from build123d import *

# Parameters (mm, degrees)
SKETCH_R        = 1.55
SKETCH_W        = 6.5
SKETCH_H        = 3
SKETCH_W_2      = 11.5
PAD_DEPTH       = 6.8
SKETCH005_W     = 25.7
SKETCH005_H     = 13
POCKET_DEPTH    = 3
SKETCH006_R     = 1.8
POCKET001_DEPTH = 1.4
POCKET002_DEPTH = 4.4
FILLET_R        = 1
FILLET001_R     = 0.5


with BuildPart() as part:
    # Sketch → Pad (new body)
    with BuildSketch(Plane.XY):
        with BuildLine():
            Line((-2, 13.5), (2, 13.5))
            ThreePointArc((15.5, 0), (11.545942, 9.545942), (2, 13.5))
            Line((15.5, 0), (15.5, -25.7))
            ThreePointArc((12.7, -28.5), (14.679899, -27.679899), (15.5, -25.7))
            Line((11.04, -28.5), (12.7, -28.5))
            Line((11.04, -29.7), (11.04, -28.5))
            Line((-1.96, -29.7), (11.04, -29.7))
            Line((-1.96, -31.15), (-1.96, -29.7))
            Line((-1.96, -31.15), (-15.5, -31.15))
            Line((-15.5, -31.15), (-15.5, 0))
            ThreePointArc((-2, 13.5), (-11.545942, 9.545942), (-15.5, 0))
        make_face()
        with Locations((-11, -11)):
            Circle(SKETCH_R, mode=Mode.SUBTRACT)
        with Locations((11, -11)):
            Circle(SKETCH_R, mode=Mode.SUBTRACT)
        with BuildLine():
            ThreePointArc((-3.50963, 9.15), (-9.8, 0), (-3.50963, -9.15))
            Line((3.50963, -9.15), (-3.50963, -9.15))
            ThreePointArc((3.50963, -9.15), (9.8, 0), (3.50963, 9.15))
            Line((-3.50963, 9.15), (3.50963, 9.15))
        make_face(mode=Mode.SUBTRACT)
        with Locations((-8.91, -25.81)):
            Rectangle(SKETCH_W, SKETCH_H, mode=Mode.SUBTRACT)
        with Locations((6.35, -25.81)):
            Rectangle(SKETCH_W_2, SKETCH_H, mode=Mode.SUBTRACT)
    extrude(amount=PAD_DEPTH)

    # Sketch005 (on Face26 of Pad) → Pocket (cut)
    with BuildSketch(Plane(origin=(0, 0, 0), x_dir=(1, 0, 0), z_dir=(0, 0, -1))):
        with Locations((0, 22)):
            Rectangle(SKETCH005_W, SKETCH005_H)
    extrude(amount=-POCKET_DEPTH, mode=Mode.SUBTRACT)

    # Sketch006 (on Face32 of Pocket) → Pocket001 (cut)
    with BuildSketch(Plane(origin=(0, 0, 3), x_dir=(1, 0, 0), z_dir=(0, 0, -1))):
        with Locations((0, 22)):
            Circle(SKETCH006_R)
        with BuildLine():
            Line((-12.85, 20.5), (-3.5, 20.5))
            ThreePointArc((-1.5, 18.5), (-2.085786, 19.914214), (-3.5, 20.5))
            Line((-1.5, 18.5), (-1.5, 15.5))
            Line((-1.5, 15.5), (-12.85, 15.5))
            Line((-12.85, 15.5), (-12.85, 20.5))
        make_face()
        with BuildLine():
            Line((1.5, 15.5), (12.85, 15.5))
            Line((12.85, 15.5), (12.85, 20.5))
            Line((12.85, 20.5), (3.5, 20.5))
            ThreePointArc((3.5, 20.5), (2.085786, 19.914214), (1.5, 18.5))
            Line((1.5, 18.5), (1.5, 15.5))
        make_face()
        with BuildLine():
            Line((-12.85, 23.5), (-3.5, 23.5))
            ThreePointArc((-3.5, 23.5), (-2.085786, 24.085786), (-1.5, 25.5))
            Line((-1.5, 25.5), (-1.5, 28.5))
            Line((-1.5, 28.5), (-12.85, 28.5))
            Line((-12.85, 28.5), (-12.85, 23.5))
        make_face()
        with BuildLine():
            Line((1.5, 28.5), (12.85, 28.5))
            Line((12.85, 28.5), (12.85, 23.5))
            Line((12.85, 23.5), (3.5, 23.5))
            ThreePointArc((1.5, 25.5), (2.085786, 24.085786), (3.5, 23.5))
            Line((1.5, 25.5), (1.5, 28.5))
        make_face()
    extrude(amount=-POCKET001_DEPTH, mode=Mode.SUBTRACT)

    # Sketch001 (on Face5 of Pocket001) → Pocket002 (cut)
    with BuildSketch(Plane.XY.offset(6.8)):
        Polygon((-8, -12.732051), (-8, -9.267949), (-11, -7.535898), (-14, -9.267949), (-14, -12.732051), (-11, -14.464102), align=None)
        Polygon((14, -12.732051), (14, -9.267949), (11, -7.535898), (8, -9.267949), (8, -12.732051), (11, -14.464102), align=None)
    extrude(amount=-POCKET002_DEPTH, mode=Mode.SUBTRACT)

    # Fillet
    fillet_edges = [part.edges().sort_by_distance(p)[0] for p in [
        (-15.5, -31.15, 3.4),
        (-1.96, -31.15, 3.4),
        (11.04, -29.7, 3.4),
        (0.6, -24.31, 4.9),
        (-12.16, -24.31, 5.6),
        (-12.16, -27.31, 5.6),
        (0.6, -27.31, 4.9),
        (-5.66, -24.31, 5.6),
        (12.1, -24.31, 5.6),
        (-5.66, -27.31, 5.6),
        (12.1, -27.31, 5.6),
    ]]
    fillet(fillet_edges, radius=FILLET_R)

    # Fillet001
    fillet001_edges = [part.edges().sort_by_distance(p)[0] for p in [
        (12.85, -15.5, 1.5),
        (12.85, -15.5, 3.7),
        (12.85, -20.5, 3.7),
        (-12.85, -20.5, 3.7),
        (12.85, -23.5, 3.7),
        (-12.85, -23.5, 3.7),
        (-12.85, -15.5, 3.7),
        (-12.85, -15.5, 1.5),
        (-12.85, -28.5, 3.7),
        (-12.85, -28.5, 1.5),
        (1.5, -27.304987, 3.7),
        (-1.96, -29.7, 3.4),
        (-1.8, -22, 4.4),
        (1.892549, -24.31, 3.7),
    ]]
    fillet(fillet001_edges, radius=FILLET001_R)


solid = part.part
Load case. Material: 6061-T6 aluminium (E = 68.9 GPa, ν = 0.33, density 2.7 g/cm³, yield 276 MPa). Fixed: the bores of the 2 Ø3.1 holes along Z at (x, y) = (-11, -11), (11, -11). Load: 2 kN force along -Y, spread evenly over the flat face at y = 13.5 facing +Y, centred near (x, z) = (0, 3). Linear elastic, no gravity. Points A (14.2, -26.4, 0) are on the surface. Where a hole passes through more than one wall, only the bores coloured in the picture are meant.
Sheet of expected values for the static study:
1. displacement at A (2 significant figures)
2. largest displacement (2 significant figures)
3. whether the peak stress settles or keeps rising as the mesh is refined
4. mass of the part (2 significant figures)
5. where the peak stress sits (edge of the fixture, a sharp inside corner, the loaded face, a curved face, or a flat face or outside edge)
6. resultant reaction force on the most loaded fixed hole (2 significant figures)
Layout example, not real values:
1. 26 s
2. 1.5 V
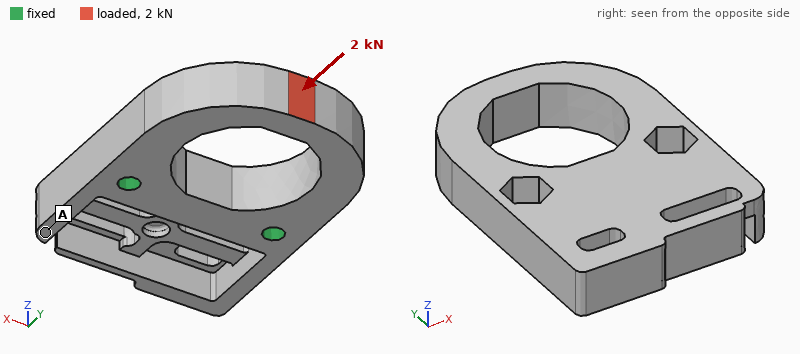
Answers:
1. 27 µm
2. 99 µm
3. keeps rising
4. 13 g
5. edge of the fixture
6. 1.1 kN
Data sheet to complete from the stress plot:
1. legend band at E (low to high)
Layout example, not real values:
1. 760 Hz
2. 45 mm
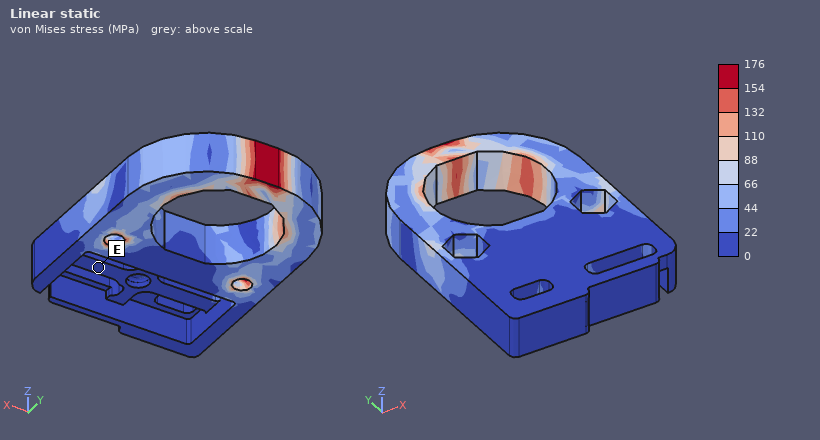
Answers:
1. 0 to 22 MPa
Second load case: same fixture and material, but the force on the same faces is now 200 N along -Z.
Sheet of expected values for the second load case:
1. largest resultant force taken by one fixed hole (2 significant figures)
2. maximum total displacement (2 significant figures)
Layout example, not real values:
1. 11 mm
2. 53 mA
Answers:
1. 100 N
2. 0.11 mm
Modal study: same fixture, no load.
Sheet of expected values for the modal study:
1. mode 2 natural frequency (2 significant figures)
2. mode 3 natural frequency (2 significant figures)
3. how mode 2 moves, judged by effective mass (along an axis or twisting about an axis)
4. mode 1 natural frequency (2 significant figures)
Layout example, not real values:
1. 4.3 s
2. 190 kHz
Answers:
1. 8300 Hz
2. 10 kHz
3. along Z
4. 4500 Hz
